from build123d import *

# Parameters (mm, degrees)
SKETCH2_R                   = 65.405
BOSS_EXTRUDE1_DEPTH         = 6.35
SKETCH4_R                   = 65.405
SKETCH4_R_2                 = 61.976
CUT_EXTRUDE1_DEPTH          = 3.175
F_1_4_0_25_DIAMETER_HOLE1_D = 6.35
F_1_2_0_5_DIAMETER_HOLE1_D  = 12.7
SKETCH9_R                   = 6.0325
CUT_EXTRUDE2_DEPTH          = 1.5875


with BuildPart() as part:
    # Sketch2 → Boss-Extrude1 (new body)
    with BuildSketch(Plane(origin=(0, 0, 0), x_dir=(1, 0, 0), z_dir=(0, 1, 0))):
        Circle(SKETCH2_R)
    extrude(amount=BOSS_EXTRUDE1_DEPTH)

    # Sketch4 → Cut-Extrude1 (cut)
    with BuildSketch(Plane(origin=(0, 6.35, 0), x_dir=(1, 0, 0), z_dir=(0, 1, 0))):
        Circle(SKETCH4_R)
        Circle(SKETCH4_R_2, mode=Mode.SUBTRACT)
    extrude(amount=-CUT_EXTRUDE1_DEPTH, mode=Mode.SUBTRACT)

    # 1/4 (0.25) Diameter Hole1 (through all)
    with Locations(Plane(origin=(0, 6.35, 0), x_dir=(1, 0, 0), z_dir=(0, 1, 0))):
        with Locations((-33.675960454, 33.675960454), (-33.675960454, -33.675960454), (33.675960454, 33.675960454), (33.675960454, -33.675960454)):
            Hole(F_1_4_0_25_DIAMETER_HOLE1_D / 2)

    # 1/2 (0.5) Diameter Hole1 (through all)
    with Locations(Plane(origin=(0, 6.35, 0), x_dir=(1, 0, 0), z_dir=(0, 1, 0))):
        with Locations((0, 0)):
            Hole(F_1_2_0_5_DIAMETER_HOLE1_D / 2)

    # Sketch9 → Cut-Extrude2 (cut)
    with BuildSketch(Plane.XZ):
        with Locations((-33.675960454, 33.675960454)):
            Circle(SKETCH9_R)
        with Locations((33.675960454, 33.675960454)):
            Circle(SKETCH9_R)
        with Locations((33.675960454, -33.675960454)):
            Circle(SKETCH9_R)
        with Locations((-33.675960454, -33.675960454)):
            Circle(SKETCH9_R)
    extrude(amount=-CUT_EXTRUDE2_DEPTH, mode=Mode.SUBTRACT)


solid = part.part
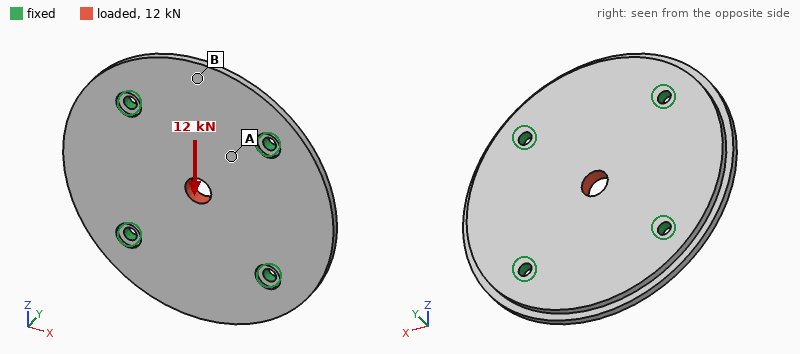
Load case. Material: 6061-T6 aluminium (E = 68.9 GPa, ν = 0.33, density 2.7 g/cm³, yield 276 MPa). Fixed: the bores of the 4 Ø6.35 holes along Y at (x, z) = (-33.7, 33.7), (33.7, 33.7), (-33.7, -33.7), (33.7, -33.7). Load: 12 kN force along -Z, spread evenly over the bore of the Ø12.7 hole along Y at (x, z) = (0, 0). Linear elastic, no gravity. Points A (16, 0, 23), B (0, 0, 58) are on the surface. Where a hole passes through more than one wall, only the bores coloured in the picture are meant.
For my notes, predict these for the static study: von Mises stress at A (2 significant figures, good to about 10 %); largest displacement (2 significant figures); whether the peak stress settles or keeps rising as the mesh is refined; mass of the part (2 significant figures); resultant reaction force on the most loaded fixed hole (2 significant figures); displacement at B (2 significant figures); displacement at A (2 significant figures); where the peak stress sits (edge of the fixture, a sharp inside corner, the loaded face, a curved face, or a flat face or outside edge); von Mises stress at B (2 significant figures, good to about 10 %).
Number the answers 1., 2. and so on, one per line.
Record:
1. 19 MPa
2. 20 µm
3. keeps rising
4. 210 g
5. 3.1 kN
6. 9.9 µm
7. 9.1 µm
8. edge of the fixture
9. 9.0 MPa
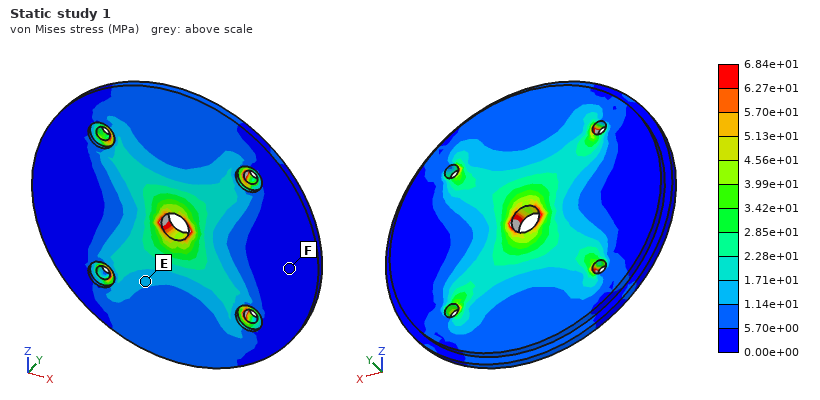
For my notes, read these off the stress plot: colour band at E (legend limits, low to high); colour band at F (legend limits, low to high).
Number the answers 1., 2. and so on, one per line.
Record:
1. 1.14e+01 to 1.71e+01 MPa
2. 0.00e+00 to 5.70e+00 MPa
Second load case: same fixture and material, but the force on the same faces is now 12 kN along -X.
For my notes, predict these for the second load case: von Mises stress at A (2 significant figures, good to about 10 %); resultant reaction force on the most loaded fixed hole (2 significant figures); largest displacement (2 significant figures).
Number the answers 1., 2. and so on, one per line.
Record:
1. 18 MPa
2. 3.1 kN
3. 20 µm
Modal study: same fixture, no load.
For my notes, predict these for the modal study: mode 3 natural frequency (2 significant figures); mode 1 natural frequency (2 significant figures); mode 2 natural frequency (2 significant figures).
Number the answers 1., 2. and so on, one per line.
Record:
1. 4200 Hz
2. 3800 Hz
3. 4200 Hz
